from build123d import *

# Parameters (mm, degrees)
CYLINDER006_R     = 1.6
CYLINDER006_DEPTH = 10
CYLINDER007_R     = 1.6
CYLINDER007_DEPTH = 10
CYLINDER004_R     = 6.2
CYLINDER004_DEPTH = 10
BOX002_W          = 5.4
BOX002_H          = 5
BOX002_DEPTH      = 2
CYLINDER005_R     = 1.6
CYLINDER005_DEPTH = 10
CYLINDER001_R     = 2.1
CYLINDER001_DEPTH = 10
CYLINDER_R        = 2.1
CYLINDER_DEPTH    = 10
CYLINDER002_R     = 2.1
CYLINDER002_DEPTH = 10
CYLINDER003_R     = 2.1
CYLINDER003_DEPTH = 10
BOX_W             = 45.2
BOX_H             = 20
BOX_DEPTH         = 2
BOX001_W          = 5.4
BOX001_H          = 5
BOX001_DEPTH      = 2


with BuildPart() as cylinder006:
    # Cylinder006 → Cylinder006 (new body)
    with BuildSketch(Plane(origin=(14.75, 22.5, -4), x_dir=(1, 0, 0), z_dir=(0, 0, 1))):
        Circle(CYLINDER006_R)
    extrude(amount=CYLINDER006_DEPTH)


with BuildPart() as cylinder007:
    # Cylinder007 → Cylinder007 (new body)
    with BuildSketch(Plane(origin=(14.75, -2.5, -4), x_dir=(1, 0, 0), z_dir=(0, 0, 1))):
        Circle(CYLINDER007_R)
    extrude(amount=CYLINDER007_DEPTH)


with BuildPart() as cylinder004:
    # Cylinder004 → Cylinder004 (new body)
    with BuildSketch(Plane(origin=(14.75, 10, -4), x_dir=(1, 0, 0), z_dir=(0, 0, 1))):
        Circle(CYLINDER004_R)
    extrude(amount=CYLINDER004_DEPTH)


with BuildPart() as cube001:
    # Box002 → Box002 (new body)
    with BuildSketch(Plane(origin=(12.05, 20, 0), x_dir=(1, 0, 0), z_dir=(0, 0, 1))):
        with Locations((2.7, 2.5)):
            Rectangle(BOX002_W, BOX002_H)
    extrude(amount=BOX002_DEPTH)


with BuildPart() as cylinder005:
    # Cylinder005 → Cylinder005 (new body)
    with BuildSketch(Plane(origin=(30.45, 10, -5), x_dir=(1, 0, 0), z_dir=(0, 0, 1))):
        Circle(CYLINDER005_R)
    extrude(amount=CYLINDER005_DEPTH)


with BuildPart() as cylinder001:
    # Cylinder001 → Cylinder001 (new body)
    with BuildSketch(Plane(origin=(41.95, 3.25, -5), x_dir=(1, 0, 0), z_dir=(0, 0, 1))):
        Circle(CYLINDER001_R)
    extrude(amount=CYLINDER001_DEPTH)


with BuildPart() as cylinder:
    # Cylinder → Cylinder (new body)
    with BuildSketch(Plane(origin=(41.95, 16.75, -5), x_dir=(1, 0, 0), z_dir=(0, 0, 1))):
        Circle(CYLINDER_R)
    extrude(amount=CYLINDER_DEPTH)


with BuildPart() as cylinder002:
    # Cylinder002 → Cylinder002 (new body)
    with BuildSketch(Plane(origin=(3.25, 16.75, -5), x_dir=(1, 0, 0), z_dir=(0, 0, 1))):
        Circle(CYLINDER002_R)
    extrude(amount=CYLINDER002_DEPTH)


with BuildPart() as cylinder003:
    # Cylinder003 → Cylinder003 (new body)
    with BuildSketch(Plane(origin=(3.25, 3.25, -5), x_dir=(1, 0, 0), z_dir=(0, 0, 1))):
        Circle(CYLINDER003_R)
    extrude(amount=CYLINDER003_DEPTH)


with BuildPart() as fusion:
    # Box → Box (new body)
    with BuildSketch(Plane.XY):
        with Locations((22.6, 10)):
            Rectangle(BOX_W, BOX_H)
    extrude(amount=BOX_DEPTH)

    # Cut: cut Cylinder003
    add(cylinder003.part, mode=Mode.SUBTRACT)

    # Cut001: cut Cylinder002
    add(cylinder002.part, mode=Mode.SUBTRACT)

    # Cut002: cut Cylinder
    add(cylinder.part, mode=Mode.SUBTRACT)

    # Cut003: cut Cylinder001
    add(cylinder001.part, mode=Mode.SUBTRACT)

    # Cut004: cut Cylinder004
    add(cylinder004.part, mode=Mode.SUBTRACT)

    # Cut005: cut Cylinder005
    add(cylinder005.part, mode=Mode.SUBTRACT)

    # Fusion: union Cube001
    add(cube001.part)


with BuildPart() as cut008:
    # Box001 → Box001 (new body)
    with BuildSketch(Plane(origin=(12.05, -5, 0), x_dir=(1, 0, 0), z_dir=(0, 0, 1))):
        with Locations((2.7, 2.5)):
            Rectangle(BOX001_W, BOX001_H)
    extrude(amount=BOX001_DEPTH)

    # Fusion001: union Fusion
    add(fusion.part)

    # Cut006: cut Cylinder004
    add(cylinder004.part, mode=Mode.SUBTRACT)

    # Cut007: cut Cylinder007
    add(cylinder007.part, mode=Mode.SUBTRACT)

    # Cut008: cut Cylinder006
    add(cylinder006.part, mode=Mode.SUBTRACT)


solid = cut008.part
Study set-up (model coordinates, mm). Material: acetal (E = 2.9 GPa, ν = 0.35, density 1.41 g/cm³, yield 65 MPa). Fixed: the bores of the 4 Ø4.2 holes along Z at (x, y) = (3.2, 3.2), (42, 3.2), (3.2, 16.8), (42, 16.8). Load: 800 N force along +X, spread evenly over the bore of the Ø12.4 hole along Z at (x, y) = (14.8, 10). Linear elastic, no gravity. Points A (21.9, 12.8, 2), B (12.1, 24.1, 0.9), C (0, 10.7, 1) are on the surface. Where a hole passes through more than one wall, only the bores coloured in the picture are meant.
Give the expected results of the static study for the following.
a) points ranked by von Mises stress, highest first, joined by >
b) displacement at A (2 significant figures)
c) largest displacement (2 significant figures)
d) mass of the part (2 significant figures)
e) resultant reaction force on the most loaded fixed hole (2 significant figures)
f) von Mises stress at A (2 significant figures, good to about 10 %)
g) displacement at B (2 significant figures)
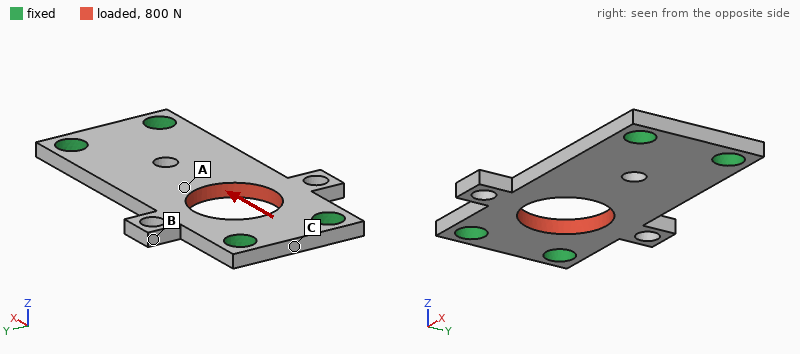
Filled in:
A > C > B
61 µm
68 µm
2.1 g
260 N
11 MPa
33 µm
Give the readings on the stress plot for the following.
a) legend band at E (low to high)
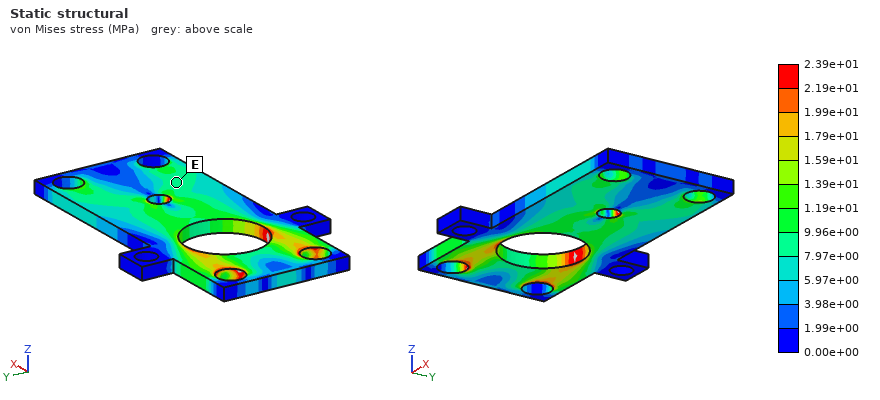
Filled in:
7.97e+00 to 9.96e+00 MPa
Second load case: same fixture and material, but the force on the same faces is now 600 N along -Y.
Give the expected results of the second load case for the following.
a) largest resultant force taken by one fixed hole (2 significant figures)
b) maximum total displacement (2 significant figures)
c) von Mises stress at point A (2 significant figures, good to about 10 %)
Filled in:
230 N
0.24 mm
10 MPa
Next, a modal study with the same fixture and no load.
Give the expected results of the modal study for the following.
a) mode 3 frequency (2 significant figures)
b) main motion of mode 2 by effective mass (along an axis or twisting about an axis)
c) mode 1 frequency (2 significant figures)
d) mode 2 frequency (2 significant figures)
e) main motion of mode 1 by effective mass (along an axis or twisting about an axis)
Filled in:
4600 Hz
twisting about X
2200 Hz
2800 Hz
along Z
